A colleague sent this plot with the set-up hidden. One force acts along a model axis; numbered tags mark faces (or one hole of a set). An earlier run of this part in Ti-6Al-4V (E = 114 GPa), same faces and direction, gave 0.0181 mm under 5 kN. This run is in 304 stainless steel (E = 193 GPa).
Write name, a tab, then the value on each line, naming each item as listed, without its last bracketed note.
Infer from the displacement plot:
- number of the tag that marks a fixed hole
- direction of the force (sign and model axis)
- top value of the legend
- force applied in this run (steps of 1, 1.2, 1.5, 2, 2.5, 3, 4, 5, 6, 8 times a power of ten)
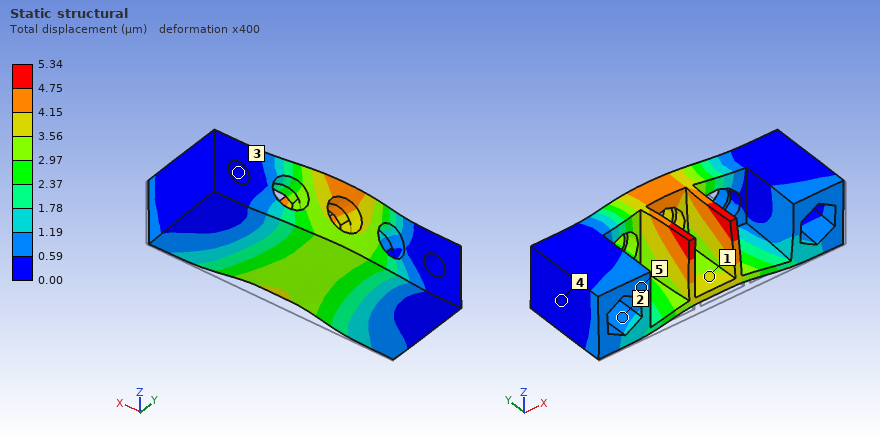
number of the tag that marks a fixed hole	3
direction of the force	+Y
top value of the legend	5.34 µm
force applied in this run	2.5 kN
